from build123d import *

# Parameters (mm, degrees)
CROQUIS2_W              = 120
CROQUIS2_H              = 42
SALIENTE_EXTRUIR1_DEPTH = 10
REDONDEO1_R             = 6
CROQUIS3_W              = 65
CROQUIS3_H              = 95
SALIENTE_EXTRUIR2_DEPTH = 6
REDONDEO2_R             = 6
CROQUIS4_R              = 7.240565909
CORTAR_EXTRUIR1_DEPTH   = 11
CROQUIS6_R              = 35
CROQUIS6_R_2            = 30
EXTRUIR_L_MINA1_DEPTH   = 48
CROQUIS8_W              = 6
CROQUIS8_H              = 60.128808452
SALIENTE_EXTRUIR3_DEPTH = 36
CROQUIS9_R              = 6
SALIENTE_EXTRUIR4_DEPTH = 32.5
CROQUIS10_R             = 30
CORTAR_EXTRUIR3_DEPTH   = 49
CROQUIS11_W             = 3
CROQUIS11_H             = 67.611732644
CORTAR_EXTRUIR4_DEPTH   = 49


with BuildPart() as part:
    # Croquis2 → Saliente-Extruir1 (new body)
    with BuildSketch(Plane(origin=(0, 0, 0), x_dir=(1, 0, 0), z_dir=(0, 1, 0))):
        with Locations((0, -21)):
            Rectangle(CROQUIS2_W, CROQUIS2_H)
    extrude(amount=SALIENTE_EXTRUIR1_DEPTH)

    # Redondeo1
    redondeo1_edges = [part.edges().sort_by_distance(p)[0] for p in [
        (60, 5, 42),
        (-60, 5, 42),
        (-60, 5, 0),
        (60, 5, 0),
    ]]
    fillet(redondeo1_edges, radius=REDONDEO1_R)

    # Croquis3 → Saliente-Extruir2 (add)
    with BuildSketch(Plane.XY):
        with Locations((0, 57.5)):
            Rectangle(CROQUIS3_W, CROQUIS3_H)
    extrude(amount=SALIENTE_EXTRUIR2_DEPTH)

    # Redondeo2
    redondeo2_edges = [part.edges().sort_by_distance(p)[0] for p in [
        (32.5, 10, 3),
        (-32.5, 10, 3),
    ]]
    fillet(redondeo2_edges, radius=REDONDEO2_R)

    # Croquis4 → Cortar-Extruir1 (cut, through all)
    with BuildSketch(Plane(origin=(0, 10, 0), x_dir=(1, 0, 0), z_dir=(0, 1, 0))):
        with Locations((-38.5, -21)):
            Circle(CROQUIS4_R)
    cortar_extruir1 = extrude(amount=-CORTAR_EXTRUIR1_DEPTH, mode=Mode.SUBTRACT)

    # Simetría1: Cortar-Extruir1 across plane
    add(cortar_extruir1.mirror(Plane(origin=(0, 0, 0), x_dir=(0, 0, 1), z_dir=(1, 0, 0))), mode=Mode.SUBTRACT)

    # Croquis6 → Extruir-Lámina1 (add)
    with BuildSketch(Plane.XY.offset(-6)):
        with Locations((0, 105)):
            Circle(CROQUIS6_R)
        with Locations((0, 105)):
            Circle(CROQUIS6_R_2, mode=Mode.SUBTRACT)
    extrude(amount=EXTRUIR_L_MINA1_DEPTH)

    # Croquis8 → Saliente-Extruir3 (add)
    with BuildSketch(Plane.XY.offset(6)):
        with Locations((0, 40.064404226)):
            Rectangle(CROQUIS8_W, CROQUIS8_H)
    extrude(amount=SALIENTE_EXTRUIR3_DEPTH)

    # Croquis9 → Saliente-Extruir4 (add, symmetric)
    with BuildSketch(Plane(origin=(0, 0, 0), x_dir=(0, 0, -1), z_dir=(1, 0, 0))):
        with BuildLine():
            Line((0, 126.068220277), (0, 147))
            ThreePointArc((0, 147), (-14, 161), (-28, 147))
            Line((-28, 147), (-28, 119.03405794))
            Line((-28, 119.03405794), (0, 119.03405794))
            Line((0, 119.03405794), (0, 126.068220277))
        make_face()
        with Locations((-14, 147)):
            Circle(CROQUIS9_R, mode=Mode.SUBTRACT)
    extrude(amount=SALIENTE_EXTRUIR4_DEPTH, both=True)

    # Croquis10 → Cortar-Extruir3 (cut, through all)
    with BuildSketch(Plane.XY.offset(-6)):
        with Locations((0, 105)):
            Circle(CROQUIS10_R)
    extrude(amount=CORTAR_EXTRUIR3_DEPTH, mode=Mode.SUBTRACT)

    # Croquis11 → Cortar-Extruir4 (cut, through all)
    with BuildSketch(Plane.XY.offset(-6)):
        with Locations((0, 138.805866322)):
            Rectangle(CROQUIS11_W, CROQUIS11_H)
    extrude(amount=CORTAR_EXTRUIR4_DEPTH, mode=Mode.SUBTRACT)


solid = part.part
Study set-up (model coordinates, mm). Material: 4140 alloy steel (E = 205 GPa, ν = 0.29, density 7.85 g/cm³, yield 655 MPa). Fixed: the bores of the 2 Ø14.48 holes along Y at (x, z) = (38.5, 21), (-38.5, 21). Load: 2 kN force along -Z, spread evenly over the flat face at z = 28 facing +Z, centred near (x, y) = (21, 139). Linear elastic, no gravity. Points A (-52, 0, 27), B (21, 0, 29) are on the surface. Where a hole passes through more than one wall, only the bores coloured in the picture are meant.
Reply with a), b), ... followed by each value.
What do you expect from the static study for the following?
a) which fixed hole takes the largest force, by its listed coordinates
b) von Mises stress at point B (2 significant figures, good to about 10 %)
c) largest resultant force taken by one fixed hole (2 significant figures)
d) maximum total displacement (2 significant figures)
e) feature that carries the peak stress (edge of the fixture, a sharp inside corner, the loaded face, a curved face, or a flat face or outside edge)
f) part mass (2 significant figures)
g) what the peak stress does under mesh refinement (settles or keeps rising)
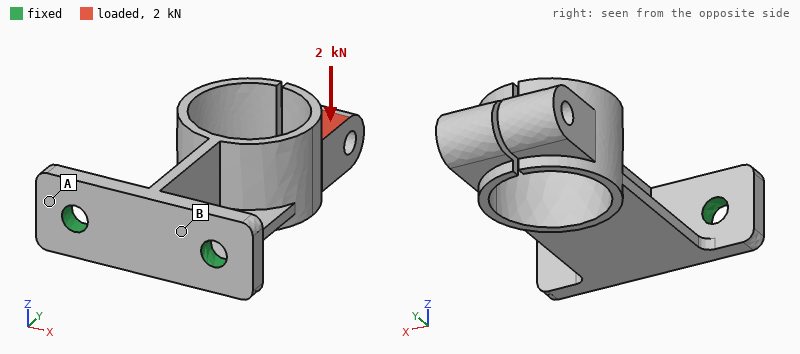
a) (38.5, 21)
b) 73 MPa
c) 1.7 kN
d) 1.4 mm
e) a sharp inside corner
f) 1.3 kg
g) keeps rising
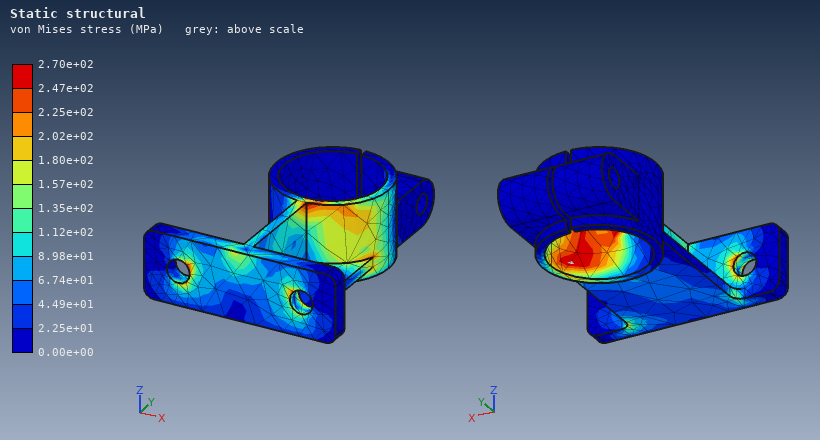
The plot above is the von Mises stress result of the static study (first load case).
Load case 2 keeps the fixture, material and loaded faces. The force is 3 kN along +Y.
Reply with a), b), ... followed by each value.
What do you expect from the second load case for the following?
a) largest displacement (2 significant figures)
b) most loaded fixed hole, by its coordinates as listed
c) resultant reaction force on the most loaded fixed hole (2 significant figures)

a) 0.69 mm
b) (38.5, 21)
c) 2.5 kN
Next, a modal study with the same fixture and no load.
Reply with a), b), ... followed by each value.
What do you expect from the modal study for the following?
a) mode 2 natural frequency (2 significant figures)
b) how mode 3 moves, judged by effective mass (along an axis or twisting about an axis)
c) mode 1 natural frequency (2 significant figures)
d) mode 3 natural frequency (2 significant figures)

a) 360 Hz
b) along Z
c) 350 Hz
d) 440 Hz
